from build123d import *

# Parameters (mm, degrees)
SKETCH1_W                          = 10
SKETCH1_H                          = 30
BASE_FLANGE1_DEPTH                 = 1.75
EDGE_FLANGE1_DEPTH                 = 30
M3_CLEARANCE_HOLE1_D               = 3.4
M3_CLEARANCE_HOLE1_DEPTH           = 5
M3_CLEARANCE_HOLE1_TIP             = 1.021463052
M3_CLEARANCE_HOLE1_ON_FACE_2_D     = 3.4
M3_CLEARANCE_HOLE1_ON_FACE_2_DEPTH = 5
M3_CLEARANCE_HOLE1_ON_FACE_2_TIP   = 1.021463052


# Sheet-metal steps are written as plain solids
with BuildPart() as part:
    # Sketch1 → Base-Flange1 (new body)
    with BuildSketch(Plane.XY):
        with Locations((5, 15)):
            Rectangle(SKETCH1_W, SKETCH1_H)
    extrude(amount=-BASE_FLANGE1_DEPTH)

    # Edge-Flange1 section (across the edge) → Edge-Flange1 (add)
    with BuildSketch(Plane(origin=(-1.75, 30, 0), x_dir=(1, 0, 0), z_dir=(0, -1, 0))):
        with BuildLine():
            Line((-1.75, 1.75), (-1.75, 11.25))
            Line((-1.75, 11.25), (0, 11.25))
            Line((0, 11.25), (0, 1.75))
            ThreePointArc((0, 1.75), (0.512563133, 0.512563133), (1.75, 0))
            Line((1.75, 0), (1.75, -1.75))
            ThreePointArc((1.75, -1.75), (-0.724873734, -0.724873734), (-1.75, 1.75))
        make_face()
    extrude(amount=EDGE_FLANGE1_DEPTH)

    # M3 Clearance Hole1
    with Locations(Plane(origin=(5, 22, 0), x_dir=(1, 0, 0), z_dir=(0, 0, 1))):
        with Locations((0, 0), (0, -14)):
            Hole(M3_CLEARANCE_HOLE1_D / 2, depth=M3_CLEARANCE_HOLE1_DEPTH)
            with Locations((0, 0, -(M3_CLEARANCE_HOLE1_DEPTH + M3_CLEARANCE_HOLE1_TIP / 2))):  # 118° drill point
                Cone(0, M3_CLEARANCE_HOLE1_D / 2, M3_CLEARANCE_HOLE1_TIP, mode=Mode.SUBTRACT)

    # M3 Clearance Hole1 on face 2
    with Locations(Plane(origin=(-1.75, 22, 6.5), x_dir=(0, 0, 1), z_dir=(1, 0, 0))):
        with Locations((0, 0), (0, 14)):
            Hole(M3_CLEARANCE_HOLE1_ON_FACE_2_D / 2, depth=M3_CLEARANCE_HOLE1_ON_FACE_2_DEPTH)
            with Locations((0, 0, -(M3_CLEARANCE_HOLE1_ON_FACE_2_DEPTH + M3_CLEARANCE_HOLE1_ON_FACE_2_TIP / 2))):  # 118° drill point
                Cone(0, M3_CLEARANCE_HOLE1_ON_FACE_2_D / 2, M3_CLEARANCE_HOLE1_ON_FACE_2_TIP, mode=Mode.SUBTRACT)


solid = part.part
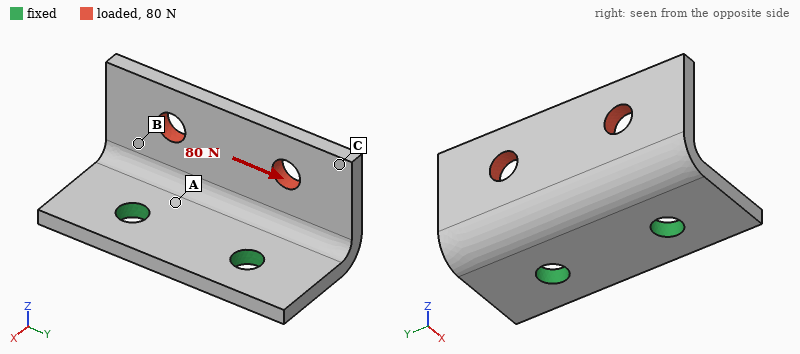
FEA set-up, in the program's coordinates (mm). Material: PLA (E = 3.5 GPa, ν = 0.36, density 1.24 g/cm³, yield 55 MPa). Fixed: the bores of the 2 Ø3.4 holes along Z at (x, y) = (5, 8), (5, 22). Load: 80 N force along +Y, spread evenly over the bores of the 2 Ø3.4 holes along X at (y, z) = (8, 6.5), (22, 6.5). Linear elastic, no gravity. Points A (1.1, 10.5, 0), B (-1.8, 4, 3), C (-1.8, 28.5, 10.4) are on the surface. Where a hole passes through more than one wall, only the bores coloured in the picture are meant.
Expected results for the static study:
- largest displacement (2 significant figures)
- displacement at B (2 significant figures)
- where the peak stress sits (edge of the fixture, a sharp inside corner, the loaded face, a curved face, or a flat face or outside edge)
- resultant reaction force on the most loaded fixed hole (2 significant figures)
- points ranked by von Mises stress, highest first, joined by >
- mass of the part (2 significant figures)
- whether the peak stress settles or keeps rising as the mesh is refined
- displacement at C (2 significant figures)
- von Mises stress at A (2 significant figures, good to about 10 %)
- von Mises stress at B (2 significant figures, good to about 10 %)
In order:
0.34 mm
0.16 mm
edge of the fixture
63 N
A > B > C
1.5 g
keeps rising
0.30 mm
14 MPa
7.4 MPa
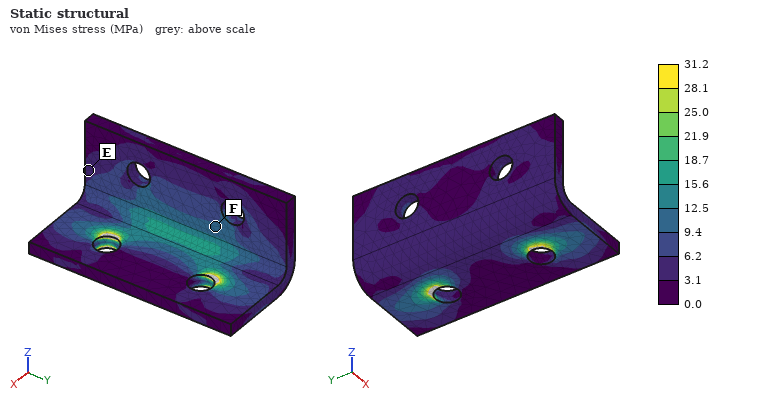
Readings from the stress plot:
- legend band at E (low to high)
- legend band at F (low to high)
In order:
3.1 to 6.2 MPa
9.4 to 12.5 MPa
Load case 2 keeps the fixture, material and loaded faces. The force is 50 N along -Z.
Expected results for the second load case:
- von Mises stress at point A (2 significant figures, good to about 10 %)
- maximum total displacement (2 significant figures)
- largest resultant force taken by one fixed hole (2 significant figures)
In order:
12 MPa
0.35 mm
25 N
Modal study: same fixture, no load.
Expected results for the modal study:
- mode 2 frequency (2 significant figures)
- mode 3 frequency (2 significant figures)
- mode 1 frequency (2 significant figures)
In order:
2600 Hz
4700 Hz
1800 Hz
